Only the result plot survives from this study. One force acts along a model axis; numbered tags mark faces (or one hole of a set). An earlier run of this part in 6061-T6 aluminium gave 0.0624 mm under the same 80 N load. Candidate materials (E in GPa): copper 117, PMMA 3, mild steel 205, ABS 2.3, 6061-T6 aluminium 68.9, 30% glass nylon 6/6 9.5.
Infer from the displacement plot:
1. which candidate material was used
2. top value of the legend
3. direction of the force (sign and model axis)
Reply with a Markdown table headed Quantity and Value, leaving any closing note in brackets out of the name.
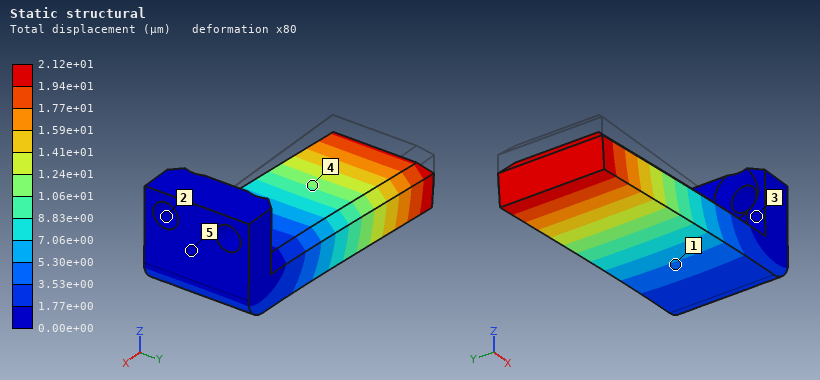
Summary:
| Quantity | Value |
|---|---|
| which candidate material was used | mild steel |
| top value of the legend | 2.12e+01 µm |
| direction of the force | -Z |
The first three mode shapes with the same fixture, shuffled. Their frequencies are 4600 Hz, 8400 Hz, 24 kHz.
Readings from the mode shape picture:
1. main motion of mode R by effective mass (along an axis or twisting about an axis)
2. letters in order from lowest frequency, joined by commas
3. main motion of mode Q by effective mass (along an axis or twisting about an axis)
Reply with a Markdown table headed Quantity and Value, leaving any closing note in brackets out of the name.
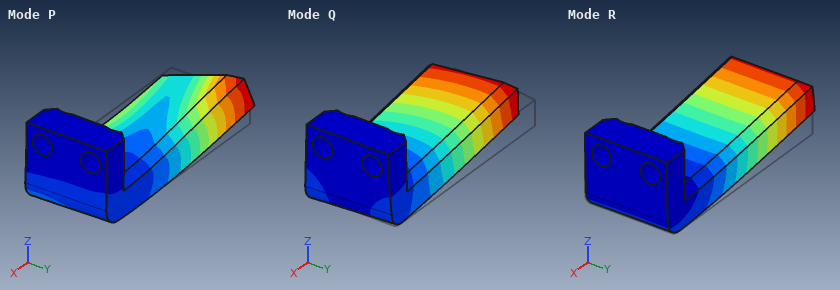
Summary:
| Quantity | Value |
|---|---|
| main motion of mode R by effective mass | along Z |
| letters in order from lowest frequency, joined by commas | R, Q, P |
| main motion of mode Q by effective mass | along Y |
